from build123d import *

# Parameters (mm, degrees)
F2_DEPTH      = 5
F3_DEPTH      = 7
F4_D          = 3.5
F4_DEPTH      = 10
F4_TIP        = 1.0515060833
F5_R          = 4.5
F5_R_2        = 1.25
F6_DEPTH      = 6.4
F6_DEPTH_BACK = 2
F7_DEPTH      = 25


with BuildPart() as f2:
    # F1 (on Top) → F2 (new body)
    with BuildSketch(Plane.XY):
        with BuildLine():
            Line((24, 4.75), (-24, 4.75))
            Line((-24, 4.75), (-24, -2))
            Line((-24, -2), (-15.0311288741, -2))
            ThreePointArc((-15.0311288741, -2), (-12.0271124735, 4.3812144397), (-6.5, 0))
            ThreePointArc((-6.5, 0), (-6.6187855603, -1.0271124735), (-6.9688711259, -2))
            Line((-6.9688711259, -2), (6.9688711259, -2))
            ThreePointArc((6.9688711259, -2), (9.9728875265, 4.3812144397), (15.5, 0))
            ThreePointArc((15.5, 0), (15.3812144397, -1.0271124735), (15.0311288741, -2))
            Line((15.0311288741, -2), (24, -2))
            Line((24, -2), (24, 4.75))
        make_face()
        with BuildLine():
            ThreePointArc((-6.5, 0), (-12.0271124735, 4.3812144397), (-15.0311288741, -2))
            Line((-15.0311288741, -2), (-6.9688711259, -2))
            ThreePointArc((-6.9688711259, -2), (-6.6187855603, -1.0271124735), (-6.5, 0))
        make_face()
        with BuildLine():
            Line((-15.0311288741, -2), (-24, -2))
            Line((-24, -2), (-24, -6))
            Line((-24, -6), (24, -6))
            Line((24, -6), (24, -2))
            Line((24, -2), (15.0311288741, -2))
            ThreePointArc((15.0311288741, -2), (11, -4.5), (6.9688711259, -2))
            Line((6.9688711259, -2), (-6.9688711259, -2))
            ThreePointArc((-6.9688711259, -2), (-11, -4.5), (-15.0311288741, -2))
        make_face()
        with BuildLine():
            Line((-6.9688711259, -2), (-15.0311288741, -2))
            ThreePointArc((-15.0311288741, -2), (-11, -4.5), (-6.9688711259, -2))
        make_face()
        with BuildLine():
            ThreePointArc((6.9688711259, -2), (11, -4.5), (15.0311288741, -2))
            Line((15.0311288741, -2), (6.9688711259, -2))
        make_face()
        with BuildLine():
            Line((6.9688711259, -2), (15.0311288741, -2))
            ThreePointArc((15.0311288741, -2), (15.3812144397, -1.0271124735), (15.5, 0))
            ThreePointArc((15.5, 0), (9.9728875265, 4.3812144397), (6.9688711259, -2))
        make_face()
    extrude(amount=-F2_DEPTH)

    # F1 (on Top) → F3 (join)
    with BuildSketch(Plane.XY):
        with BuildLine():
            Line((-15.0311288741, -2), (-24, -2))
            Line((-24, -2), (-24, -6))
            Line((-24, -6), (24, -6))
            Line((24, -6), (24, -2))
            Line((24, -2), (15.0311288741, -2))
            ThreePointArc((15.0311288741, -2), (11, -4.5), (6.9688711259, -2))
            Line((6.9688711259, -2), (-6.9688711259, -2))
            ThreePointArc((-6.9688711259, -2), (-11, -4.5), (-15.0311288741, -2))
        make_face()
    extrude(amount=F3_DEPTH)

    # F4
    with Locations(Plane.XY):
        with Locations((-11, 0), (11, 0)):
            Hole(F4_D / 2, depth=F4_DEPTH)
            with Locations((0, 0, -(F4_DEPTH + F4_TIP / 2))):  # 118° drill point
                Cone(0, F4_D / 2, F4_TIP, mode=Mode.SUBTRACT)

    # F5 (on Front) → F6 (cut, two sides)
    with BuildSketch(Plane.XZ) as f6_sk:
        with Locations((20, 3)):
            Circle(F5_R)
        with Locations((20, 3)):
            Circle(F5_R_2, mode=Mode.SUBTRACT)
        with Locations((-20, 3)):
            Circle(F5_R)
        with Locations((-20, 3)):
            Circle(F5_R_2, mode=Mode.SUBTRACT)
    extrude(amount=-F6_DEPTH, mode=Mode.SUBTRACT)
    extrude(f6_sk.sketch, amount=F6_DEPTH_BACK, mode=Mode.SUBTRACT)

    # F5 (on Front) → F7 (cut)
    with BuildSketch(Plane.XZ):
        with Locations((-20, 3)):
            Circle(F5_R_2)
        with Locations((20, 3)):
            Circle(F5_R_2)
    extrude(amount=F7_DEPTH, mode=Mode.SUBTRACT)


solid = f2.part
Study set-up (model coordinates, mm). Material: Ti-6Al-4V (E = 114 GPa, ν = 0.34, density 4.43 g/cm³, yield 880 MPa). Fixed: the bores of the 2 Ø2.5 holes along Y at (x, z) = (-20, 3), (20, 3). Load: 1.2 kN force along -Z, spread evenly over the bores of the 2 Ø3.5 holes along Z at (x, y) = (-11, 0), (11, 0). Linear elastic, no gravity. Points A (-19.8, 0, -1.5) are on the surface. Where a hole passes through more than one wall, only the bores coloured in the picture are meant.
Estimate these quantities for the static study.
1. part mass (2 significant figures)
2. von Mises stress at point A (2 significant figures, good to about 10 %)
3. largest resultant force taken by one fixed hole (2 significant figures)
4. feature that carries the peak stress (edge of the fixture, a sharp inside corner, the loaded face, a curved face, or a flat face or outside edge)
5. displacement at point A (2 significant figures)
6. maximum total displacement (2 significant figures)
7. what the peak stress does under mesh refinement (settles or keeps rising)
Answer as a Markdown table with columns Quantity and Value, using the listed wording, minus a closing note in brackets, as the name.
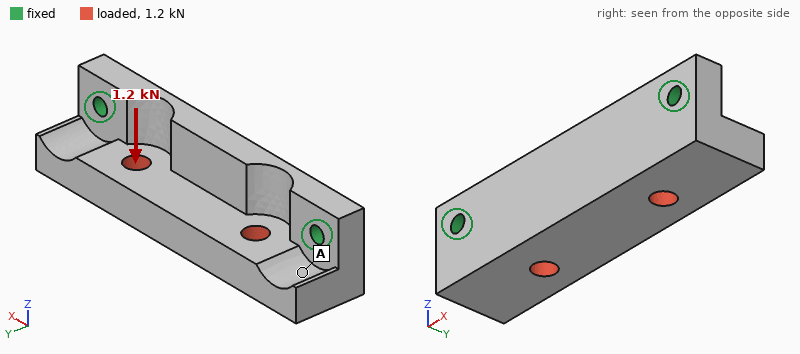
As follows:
| Quantity | Value |
|---|---|
| part mass | 15 g |
| von Mises stress at point A | 23 MPa |
| largest resultant force taken by one fixed hole | 690 N |
| feature that carries the peak stress | edge of the fixture |
| displacement at point A | 9.3 µm |
| maximum total displacement | 41 µm |
| what the peak stress does under mesh refinement | keeps rising |
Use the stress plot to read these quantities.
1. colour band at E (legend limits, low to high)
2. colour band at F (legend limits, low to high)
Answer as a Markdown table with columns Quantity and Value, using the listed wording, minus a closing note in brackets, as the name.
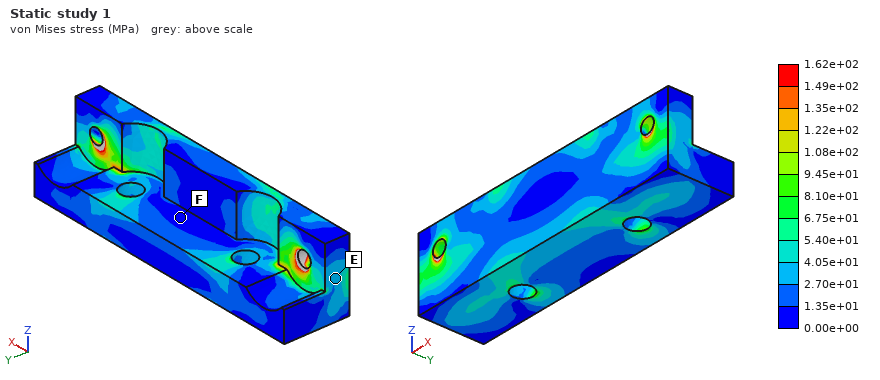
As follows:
| Quantity | Value |
|---|---|
| colour band at E | 2.70e+01 to 4.05e+01 MPa |
| colour band at F | 0.00e+00 to 1.35e+01 MPa |
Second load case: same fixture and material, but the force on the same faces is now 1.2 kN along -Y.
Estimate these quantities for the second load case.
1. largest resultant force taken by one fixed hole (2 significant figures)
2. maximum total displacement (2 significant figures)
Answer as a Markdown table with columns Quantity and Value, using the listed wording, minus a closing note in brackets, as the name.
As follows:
| Quantity | Value |
|---|---|
| largest resultant force taken by one fixed hole | 620 N |
| maximum total displacement | 31 µm |
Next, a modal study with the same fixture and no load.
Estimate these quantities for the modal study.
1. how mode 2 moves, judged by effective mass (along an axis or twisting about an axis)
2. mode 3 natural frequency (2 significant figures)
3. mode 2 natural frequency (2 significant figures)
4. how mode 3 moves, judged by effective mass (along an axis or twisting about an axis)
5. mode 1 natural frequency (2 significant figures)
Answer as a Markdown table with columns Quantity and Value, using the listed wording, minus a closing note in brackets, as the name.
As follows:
| Quantity | Value |
|---|---|
| how mode 2 moves, judged by effective mass | along Y |
| mode 3 natural frequency | 19 kHz |
| mode 2 natural frequency | 15 kHz |
| how mode 3 moves, judged by effective mass | along Z |
| mode 1 natural frequency | 10 kHz |
